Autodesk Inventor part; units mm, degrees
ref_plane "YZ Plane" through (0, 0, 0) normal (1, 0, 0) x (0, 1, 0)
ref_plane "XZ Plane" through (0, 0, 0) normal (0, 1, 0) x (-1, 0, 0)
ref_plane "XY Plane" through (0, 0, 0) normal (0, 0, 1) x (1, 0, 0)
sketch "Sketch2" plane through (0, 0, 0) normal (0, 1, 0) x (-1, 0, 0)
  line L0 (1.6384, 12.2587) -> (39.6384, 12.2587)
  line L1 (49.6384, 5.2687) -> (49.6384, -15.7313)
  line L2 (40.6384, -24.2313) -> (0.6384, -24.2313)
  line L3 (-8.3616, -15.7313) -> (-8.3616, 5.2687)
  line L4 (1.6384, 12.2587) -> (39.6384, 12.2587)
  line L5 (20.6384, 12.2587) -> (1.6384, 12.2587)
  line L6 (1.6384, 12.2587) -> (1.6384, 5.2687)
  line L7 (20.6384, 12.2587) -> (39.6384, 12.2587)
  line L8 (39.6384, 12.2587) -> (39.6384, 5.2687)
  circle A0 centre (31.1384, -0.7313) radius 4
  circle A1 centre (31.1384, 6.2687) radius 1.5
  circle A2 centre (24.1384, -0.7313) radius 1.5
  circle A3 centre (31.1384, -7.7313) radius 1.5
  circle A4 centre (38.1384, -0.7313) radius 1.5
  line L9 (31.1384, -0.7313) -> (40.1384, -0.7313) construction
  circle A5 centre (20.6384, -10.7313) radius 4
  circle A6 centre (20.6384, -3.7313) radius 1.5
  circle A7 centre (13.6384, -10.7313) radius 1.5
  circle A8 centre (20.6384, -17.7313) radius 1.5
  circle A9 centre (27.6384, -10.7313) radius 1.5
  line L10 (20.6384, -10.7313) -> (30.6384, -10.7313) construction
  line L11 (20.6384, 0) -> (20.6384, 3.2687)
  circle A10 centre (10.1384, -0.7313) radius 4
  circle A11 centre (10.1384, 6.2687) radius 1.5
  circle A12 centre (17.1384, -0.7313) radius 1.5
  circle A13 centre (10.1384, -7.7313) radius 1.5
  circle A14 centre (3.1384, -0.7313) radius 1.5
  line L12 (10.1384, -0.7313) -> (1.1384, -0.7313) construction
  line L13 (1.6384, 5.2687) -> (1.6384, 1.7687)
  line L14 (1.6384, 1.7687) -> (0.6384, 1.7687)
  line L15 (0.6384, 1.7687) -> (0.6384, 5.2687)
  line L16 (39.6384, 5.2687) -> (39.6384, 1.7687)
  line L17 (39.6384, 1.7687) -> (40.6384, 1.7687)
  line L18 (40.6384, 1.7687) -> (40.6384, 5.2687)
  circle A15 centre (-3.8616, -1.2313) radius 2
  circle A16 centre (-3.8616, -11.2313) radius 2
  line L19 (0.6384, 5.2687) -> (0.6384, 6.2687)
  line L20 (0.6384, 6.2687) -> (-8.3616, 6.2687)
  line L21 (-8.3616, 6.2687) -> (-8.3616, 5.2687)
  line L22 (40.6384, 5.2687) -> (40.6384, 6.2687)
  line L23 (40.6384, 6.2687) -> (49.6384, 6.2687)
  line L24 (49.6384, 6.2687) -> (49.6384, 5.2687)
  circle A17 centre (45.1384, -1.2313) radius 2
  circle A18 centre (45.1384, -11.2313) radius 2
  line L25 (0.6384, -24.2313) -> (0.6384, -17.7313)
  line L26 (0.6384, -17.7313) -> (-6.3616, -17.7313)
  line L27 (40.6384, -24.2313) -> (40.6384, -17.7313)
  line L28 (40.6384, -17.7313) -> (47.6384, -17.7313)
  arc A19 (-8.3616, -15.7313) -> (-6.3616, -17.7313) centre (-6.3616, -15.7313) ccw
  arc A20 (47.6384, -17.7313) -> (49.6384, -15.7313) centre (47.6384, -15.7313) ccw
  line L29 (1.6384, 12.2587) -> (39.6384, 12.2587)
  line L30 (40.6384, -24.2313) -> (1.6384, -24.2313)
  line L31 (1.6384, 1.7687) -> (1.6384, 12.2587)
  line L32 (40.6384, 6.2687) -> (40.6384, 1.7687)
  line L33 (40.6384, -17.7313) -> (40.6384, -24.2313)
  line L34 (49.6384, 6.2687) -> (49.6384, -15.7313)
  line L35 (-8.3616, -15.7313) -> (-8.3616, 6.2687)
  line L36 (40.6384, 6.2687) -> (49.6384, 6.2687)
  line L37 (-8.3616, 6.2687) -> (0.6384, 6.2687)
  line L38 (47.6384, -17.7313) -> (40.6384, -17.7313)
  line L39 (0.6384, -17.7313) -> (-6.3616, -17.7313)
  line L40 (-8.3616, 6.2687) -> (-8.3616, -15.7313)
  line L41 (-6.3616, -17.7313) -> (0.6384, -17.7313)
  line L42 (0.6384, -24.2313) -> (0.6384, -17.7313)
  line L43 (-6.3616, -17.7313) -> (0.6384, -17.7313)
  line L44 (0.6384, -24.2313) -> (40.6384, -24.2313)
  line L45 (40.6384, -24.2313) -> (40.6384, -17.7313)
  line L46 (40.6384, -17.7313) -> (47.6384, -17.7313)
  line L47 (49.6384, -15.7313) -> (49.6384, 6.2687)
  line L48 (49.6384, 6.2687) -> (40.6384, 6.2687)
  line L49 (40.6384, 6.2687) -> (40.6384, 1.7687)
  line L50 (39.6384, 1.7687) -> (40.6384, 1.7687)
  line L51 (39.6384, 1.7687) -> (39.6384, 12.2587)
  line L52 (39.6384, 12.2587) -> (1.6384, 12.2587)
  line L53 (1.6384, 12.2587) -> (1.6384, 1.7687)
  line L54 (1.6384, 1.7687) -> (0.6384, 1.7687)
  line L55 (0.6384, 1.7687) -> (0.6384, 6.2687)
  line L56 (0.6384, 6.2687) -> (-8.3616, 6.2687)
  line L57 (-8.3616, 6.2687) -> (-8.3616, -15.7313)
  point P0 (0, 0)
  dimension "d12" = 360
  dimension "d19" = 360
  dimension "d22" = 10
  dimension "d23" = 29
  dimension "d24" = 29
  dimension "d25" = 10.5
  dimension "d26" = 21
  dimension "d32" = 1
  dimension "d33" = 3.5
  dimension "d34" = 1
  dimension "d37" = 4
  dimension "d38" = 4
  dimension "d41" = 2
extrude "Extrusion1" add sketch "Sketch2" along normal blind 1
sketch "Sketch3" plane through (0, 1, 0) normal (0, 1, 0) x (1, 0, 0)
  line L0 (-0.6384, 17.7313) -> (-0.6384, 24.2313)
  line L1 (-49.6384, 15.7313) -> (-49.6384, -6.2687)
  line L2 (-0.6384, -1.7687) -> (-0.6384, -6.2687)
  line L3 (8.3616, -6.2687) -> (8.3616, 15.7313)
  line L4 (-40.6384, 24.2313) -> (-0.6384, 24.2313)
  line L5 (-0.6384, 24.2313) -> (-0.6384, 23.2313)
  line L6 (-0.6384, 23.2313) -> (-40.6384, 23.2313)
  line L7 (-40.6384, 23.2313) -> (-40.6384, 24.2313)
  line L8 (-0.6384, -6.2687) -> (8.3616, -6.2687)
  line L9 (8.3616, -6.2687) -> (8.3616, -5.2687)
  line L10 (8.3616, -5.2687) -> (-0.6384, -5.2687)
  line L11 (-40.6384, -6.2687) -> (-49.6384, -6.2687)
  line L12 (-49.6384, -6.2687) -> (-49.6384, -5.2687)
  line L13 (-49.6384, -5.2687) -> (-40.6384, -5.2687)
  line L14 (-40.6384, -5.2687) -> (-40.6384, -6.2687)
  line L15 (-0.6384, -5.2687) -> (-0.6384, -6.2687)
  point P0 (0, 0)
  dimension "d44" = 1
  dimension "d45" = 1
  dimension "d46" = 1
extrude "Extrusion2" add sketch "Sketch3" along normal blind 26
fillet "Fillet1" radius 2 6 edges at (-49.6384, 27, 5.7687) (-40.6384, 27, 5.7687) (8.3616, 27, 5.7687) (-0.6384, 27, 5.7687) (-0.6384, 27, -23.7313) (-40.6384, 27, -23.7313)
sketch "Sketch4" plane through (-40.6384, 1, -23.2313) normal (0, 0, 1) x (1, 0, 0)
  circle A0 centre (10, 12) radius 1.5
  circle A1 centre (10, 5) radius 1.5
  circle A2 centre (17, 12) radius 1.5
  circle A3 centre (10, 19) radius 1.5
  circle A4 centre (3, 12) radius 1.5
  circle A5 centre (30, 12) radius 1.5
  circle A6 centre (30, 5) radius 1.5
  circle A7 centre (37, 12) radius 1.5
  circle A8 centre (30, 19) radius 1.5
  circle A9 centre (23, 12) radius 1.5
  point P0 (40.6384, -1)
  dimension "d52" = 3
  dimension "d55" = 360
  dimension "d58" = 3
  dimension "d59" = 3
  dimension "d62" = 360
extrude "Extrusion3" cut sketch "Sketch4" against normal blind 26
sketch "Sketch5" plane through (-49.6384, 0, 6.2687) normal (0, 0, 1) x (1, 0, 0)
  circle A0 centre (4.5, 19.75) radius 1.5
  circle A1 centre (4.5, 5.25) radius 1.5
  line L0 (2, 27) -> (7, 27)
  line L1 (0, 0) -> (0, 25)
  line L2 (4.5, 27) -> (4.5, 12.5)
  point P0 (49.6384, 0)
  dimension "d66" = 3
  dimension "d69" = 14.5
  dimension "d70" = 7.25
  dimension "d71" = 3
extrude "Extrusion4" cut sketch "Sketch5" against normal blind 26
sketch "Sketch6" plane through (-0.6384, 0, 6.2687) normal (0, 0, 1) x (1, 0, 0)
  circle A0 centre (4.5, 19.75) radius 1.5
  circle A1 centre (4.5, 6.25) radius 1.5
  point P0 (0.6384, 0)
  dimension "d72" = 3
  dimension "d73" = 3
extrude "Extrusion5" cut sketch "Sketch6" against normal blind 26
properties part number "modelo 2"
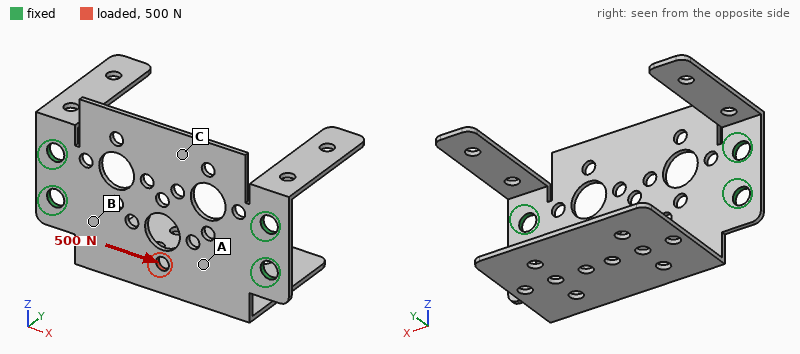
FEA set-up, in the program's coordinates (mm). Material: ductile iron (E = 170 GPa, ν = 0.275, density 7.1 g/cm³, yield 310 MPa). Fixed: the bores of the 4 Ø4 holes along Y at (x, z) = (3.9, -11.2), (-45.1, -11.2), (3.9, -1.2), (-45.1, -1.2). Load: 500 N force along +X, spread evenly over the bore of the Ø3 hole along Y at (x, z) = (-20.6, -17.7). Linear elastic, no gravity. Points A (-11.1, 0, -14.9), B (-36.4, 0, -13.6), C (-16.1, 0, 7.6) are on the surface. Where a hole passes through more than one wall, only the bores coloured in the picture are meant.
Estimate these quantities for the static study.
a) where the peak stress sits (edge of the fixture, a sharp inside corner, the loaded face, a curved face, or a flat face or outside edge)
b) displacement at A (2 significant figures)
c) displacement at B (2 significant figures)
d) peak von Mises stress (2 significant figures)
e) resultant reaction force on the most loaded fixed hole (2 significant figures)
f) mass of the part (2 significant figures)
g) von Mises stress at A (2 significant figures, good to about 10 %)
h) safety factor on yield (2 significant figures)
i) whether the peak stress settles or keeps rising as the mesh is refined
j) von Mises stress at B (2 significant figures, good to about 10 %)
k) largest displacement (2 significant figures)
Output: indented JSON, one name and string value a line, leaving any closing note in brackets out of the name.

{
  "where the peak stress sits": "the loaded face",
  "displacement at A": "2.2 µm",
  "displacement at B": "1.1 µm",
  "peak von Mises stress": "100 MPa",
  "resultant reaction force on the most loaded fixed hole": "210 N",
  "mass of the part": "21 g",
  "von Mises stress at A": "27 MPa",
  "safety factor on yield": "3.1",
  "whether the peak stress settles or keeps rising as the mesh is refined": "settles",
  "von Mises stress at B": "23 MPa",
  "largest displacement": "4.3 µm"
}
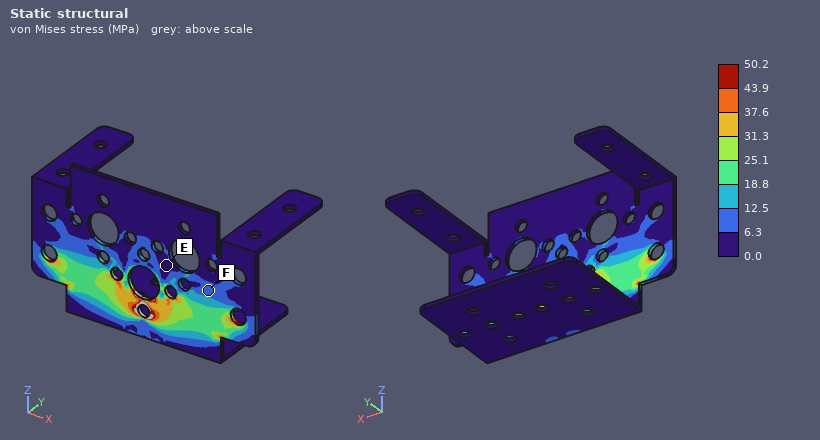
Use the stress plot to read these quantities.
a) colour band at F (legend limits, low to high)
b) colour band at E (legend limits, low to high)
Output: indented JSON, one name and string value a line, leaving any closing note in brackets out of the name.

{
  "colour band at F": "6.3 to 12.5 MPa",
  "colour band at E": "0.0 to 6.3 MPa"
}
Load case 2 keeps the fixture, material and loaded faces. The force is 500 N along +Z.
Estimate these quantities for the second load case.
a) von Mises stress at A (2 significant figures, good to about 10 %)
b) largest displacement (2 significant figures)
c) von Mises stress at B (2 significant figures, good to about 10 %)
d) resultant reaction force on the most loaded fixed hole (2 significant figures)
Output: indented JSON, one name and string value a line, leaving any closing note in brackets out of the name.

{
  "von Mises stress at A": "22 MPa",
  "largest displacement": "9.3 µm",
  "von Mises stress at B": "19 MPa",
  "resultant reaction force on the most loaded fixed hole": "170 N"
}
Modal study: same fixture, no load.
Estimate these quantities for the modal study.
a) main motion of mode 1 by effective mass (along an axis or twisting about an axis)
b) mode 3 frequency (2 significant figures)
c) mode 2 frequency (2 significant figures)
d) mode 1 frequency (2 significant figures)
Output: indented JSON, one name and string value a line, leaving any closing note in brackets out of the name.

{
  "main motion of mode 1 by effective mass": "along Z",
  "mode 3 frequency": "870 Hz",
  "mode 2 frequency": "860 Hz",
  "mode 1 frequency": "610 Hz"
}
